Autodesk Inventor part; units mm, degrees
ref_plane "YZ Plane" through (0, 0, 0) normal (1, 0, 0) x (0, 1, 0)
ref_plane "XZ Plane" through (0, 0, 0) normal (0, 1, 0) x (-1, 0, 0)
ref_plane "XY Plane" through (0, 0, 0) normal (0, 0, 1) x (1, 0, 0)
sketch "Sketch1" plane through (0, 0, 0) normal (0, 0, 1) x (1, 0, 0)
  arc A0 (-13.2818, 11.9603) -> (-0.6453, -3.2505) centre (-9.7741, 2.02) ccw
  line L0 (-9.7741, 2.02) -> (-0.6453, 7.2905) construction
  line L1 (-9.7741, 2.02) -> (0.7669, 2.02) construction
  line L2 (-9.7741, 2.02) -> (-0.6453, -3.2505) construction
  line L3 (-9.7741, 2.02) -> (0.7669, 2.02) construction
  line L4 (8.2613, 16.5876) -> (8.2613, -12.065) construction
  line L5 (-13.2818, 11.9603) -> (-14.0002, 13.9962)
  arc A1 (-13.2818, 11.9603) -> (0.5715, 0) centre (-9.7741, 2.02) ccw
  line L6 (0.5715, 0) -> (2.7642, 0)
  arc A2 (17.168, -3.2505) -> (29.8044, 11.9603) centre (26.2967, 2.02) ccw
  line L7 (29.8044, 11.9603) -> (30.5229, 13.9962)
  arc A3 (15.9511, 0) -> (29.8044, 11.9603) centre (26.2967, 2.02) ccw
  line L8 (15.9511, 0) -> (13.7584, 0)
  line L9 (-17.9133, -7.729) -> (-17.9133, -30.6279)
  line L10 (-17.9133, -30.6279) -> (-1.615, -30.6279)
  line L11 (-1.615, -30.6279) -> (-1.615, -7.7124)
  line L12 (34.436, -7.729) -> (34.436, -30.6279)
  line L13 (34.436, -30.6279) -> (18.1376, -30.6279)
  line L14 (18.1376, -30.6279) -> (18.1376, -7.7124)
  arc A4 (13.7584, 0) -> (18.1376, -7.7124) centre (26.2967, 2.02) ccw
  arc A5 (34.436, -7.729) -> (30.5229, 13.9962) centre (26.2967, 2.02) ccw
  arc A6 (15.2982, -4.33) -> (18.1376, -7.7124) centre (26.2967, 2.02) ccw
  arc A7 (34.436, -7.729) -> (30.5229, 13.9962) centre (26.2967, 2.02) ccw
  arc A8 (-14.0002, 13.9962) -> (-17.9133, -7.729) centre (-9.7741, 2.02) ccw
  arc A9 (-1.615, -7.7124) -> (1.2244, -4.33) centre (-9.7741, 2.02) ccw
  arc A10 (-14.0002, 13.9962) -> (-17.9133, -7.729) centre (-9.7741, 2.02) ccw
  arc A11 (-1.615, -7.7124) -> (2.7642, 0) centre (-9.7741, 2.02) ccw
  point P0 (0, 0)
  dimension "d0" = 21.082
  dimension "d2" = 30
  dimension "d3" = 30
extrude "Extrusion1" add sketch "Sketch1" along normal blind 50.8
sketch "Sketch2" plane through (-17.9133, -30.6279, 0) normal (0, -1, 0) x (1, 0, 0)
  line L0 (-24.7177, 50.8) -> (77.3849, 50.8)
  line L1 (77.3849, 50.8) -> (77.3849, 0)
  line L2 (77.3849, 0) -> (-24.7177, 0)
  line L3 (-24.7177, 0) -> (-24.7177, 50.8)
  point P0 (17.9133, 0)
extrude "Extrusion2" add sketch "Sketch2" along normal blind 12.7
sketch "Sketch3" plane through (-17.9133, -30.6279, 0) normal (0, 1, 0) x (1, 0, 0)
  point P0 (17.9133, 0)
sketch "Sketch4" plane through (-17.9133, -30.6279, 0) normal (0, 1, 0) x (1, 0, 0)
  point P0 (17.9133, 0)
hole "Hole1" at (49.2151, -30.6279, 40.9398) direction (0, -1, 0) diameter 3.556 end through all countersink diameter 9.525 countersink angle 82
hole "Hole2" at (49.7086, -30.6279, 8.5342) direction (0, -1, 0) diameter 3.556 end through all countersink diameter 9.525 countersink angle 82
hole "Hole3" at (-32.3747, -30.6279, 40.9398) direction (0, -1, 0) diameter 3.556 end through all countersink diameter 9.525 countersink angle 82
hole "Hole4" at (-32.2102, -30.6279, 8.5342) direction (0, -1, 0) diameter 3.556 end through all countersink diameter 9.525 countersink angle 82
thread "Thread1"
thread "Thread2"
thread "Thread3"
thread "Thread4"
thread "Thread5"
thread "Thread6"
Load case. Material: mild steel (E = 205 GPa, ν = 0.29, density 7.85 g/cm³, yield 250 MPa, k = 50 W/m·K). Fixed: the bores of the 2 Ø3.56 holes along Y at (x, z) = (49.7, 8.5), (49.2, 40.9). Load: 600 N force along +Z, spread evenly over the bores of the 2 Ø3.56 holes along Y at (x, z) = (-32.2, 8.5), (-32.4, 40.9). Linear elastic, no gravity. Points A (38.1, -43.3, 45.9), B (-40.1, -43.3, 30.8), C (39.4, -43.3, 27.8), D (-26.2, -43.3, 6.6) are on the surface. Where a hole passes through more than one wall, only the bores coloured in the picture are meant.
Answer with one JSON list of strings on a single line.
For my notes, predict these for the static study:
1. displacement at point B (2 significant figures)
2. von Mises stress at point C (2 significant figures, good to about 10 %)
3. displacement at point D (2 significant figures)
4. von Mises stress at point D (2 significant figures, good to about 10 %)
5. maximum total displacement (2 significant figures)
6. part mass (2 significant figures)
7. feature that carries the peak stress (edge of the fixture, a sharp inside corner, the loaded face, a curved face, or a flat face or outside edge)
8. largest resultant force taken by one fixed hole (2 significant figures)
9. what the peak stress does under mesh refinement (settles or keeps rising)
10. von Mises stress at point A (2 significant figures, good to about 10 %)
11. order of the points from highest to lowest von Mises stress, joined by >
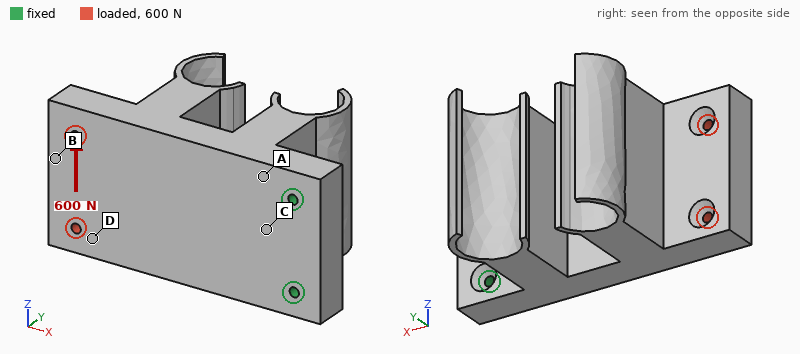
["7.0 µm", "4.4 MPa", "6.0 µm", "2.2 MPa", "7.6 µm", "870 g", "edge of the fixture", "1.5 kN", "keeps rising", "6.3 MPa", "A > C > D > B"]
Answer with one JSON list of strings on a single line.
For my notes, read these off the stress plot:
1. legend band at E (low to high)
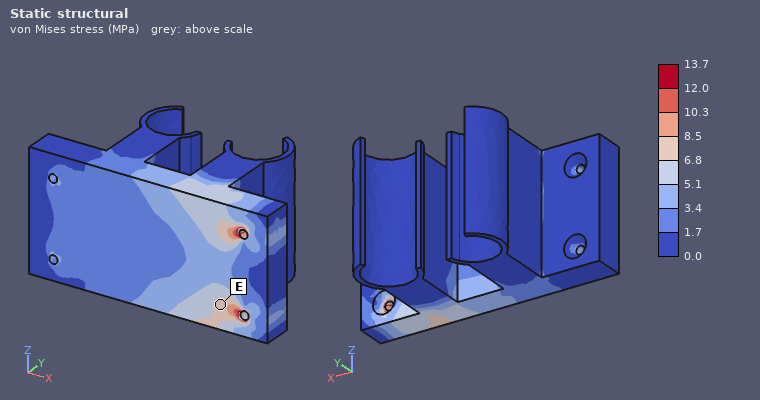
["6.8 to 8.5 MPa"]
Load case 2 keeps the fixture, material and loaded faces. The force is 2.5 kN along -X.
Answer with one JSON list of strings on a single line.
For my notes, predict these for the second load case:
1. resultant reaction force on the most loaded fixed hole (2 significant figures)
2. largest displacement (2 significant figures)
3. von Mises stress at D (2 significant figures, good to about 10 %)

["1.3 kN", "10 µm", "10 MPa"]
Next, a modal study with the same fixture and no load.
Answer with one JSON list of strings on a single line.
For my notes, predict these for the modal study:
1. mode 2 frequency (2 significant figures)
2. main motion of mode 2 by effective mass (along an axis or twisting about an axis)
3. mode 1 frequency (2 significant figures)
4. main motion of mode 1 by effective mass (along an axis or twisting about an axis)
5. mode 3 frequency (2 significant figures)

["2700 Hz", "along Z", "810 Hz", "along Y", "2900 Hz"]
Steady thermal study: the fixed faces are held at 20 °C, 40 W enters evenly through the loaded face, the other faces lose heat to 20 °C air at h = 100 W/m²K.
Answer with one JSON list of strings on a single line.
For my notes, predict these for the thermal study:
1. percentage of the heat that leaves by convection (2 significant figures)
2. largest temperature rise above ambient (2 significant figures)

["83 %", "47 K"]
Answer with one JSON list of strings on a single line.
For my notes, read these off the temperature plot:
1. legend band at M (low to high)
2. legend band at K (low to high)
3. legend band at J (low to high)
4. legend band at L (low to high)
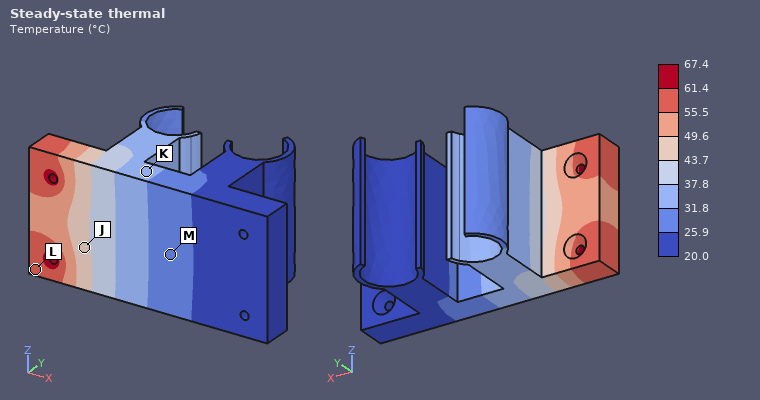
["25.9 to 31.8 °C", "31.8 to 37.8 °C", "43.7 to 49.6 °C", "55.5 to 61.4 °C"]
